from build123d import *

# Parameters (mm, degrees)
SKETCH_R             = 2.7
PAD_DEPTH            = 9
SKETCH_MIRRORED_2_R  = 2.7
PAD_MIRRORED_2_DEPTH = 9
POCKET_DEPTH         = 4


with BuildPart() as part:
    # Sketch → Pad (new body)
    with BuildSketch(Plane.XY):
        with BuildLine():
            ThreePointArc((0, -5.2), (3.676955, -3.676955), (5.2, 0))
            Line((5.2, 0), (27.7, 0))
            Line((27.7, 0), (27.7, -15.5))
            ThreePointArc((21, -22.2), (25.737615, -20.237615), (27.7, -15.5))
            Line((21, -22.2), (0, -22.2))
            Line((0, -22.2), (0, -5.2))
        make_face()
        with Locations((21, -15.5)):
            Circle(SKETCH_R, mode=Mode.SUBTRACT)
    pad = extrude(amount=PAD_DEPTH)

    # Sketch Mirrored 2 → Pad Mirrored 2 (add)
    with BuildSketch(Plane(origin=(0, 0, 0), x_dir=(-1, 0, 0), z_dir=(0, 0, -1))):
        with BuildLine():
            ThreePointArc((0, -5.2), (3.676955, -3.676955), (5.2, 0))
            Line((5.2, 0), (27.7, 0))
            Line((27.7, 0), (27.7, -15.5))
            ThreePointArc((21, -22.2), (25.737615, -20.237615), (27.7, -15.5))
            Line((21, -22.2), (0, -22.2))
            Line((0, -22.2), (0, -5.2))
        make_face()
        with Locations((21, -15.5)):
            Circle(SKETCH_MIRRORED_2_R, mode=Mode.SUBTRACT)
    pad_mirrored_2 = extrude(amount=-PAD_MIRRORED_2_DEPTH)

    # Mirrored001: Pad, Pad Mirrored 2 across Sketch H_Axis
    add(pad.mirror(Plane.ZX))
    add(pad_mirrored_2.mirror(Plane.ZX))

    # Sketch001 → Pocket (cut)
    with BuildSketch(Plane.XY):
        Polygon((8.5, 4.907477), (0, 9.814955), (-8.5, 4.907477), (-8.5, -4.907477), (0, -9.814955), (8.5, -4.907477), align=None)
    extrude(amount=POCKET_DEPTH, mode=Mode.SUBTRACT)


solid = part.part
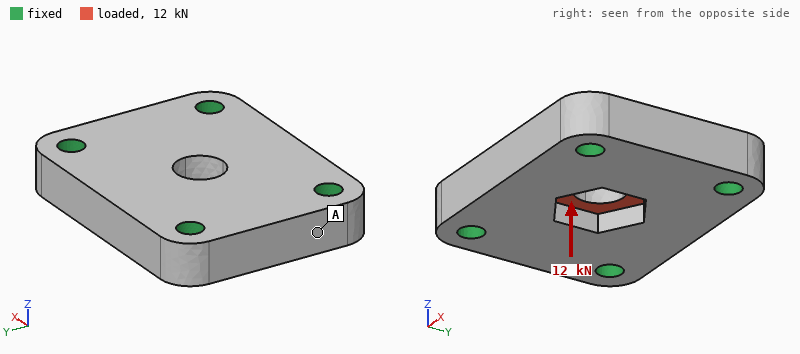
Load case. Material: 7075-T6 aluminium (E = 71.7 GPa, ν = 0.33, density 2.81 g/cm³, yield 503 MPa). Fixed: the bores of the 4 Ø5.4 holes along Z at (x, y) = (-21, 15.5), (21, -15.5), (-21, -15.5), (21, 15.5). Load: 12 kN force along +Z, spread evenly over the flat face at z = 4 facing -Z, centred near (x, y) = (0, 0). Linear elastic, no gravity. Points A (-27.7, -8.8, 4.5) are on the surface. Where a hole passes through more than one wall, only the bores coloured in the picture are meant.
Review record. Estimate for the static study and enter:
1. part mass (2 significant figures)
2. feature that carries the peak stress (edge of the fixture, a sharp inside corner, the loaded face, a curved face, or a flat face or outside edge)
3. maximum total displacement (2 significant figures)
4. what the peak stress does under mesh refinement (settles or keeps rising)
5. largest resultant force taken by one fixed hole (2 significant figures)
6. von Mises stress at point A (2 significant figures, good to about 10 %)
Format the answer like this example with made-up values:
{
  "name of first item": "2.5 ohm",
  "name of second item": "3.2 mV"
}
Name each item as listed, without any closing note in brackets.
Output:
{
  "part mass": "55 g",
  "feature that carries the peak stress": "edge of the fixture",
  "maximum total displacement": "78 µm",
  "what the peak stress does under mesh refinement": "keeps rising",
  "largest resultant force taken by one fixed hole": "3.1 kN",
  "von Mises stress at point A": "37 MPa"
}
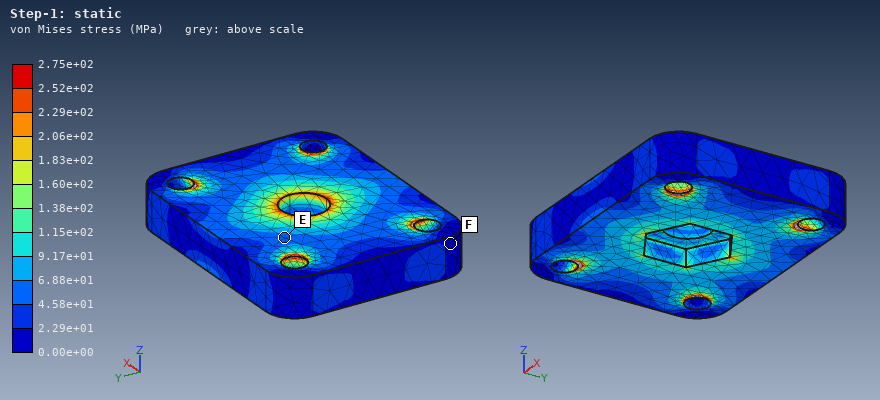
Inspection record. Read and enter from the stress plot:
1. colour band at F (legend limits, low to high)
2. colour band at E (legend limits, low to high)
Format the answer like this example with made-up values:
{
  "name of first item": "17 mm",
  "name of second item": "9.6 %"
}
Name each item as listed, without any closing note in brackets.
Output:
{
  "colour band at F": "0.00e+00 to 2.29e+01 MPa",
  "colour band at E": "4.58e+01 to 6.88e+01 MPa"
}
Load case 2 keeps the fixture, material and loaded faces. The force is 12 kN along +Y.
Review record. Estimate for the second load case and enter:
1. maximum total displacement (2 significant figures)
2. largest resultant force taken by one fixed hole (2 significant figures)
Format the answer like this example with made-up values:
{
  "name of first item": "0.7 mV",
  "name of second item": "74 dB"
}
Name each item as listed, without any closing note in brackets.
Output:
{
  "maximum total displacement": "22 µm",
  "largest resultant force taken by one fixed hole": "3.4 kN"
}
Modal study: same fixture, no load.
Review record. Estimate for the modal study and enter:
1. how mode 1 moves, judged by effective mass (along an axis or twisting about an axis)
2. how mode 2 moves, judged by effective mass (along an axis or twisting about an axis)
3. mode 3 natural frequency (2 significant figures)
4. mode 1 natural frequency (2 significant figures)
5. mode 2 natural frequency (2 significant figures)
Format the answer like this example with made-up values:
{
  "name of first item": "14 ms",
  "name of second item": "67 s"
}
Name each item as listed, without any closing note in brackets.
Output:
{
  "how mode 1 moves, judged by effective mass": "along Z",
  "how mode 2 moves, judged by effective mass": "twisting about X",
  "mode 3 natural frequency": "31 kHz",
  "mode 1 natural frequency": "20 kHz",
  "mode 2 natural frequency": "25 kHz"
}
